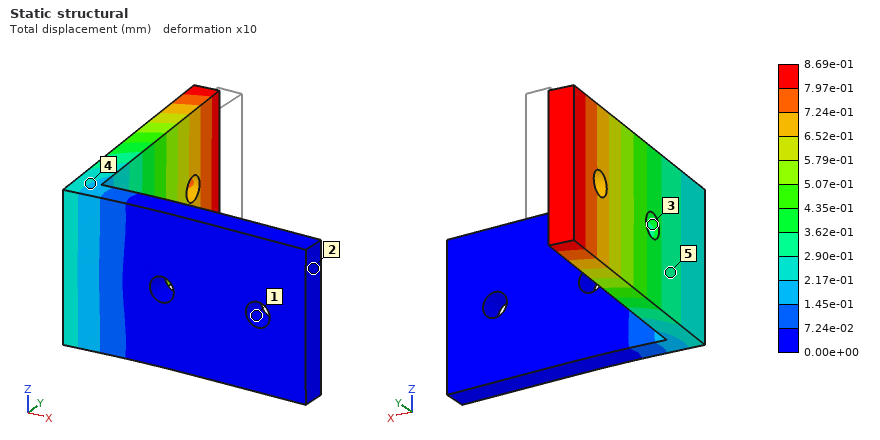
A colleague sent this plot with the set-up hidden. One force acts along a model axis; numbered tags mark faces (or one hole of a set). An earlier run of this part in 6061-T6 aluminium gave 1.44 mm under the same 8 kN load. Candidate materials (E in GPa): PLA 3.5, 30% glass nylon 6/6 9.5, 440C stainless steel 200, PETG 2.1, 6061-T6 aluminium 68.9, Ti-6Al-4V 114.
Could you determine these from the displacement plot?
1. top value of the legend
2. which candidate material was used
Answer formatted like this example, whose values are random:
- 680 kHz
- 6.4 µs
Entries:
- 8.69e-01 mm
- Ti-6Al-4V
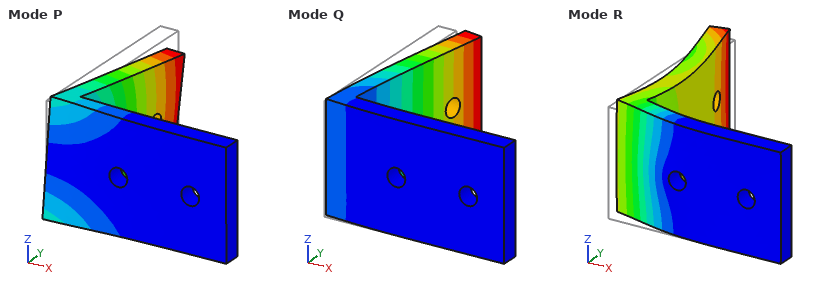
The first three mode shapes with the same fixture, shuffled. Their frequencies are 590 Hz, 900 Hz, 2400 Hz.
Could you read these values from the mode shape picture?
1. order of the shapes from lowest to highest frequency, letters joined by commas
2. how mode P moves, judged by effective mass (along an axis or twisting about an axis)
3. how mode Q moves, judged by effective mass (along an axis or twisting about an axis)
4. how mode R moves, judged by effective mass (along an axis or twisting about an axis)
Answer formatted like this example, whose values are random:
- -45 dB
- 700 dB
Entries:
- Q, P, R
- along Z
- along X
- along Y
